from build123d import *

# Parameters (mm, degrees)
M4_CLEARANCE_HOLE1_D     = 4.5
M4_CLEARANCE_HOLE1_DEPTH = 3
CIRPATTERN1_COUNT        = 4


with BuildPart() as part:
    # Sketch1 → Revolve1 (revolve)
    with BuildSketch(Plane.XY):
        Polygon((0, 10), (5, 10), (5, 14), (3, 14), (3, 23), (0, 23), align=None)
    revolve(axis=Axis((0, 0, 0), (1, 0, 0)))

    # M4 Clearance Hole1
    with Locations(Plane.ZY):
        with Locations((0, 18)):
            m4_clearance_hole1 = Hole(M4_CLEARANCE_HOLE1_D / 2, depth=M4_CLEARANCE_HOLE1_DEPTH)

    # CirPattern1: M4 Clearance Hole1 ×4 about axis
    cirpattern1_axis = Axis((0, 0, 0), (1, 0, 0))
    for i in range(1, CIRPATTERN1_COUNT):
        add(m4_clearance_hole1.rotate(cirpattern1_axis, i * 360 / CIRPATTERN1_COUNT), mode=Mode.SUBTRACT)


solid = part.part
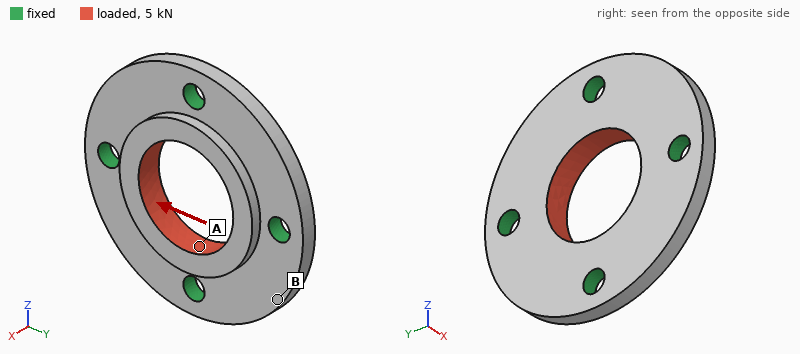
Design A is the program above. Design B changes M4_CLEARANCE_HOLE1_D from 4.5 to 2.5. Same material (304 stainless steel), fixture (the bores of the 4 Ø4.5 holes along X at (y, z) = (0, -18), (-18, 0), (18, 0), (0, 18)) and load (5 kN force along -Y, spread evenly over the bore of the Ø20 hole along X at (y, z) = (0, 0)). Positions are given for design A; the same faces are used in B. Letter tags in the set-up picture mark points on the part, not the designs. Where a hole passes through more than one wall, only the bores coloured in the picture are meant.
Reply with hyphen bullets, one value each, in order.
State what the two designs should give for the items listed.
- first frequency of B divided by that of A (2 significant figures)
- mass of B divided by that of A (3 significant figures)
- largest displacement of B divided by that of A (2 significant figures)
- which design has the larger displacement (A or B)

- 0.80
- 1.03
- 1.2
- B
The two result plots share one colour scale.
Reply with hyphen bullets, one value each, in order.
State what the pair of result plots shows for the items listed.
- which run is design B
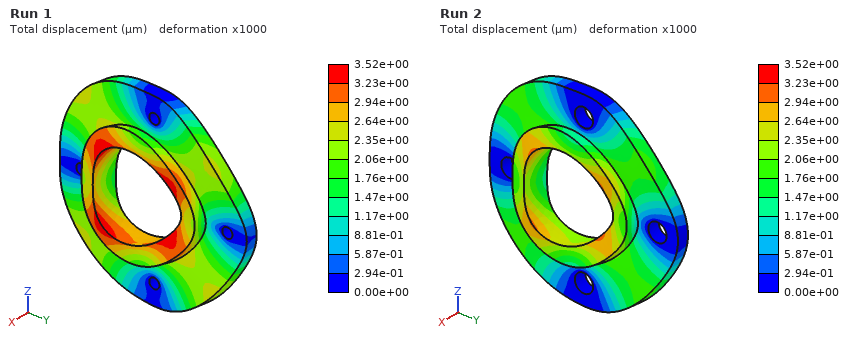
- Run 1
